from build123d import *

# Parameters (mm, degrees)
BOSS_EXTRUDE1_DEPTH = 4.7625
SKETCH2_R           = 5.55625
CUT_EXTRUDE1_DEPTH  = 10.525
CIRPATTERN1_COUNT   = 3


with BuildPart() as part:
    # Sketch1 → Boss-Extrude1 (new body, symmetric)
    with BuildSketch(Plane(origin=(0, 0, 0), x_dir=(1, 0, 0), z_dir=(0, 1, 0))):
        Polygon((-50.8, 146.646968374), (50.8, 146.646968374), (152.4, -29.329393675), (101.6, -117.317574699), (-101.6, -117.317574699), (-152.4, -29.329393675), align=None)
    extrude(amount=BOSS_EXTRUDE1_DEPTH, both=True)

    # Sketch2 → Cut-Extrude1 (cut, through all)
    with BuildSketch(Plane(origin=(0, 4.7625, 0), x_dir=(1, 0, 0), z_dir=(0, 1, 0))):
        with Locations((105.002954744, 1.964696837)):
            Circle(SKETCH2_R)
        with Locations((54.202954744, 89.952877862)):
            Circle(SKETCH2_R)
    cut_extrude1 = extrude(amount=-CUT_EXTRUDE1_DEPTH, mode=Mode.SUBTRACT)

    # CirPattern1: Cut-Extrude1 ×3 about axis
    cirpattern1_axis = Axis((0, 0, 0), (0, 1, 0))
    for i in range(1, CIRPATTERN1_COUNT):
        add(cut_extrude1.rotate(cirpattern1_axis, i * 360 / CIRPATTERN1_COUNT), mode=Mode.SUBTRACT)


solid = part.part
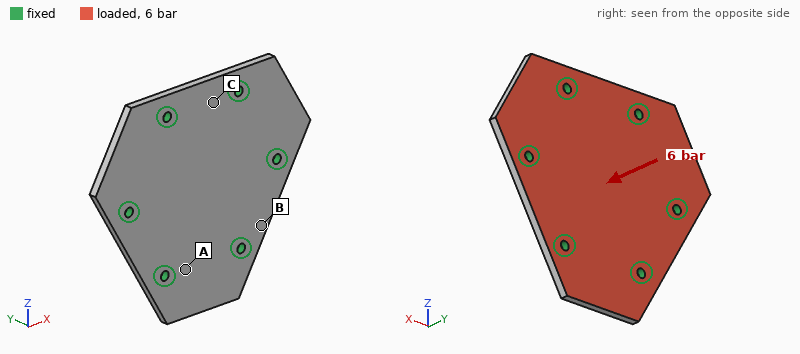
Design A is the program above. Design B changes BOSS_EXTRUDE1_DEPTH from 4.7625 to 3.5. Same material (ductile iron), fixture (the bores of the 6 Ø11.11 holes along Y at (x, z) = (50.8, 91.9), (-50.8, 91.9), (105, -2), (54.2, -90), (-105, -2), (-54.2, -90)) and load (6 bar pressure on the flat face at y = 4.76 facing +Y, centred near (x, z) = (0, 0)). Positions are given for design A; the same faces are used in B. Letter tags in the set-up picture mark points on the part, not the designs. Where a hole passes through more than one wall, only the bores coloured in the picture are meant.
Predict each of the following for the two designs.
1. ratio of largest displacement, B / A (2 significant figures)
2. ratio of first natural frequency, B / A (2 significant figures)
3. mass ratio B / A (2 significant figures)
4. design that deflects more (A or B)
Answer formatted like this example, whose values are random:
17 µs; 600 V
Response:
2.4; 0.76; 0.73; B
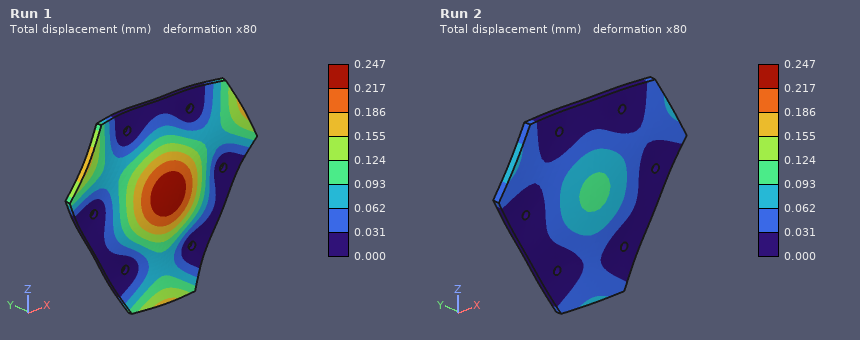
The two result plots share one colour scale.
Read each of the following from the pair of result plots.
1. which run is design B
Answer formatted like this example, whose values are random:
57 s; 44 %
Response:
Run 1
